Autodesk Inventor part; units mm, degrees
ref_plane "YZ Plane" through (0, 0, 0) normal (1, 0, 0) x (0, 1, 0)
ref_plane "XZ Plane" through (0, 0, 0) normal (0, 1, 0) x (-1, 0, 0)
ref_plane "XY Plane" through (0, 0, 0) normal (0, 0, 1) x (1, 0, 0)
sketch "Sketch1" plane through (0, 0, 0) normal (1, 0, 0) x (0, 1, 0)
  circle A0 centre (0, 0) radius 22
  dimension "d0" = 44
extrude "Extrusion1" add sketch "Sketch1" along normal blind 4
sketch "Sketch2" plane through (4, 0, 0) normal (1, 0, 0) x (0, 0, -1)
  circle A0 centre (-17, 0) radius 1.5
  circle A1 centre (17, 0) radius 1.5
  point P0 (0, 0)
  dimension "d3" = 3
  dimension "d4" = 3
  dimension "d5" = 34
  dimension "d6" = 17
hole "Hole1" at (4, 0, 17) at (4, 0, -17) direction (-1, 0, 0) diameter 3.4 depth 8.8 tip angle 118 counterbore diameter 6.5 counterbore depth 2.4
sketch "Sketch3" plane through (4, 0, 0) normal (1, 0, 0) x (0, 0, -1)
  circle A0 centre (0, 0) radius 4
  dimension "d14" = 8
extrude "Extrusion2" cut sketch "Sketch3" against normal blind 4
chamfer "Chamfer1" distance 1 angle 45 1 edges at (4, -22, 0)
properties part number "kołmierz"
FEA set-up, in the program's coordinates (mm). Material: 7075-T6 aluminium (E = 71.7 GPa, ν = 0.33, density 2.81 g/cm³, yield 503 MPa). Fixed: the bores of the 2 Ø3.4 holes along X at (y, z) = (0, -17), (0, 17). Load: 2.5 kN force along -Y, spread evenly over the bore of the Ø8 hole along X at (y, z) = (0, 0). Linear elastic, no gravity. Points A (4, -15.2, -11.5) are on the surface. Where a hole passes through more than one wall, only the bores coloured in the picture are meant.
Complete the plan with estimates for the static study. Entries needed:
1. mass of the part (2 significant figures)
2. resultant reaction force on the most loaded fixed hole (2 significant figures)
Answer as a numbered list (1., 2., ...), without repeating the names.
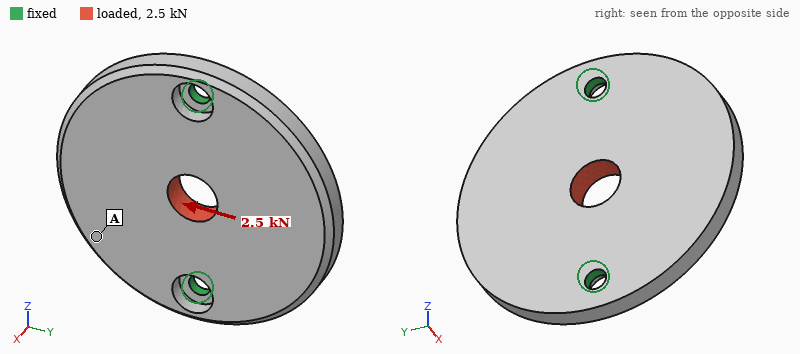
1. 16 g
2. 1.3 kN
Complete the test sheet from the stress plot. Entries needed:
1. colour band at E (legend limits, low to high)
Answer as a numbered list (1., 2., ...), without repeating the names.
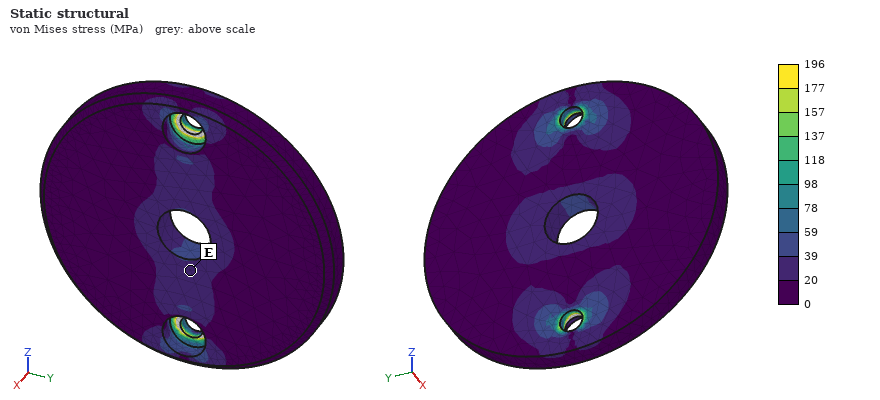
1. 20 to 39 MPa
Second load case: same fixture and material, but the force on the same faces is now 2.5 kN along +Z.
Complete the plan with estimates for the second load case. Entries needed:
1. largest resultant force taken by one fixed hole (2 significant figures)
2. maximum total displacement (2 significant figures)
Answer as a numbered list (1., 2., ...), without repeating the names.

1. 1.3 kN
2. 8.8 µm
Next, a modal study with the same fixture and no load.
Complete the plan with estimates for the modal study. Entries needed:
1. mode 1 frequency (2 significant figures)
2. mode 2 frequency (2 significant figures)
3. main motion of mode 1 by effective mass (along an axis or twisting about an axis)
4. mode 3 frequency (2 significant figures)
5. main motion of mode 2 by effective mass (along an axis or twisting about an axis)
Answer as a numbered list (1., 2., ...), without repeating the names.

1. 3300 Hz
2. 6300 Hz
3. twisting about Z
4. 12 kHz
5. along X
